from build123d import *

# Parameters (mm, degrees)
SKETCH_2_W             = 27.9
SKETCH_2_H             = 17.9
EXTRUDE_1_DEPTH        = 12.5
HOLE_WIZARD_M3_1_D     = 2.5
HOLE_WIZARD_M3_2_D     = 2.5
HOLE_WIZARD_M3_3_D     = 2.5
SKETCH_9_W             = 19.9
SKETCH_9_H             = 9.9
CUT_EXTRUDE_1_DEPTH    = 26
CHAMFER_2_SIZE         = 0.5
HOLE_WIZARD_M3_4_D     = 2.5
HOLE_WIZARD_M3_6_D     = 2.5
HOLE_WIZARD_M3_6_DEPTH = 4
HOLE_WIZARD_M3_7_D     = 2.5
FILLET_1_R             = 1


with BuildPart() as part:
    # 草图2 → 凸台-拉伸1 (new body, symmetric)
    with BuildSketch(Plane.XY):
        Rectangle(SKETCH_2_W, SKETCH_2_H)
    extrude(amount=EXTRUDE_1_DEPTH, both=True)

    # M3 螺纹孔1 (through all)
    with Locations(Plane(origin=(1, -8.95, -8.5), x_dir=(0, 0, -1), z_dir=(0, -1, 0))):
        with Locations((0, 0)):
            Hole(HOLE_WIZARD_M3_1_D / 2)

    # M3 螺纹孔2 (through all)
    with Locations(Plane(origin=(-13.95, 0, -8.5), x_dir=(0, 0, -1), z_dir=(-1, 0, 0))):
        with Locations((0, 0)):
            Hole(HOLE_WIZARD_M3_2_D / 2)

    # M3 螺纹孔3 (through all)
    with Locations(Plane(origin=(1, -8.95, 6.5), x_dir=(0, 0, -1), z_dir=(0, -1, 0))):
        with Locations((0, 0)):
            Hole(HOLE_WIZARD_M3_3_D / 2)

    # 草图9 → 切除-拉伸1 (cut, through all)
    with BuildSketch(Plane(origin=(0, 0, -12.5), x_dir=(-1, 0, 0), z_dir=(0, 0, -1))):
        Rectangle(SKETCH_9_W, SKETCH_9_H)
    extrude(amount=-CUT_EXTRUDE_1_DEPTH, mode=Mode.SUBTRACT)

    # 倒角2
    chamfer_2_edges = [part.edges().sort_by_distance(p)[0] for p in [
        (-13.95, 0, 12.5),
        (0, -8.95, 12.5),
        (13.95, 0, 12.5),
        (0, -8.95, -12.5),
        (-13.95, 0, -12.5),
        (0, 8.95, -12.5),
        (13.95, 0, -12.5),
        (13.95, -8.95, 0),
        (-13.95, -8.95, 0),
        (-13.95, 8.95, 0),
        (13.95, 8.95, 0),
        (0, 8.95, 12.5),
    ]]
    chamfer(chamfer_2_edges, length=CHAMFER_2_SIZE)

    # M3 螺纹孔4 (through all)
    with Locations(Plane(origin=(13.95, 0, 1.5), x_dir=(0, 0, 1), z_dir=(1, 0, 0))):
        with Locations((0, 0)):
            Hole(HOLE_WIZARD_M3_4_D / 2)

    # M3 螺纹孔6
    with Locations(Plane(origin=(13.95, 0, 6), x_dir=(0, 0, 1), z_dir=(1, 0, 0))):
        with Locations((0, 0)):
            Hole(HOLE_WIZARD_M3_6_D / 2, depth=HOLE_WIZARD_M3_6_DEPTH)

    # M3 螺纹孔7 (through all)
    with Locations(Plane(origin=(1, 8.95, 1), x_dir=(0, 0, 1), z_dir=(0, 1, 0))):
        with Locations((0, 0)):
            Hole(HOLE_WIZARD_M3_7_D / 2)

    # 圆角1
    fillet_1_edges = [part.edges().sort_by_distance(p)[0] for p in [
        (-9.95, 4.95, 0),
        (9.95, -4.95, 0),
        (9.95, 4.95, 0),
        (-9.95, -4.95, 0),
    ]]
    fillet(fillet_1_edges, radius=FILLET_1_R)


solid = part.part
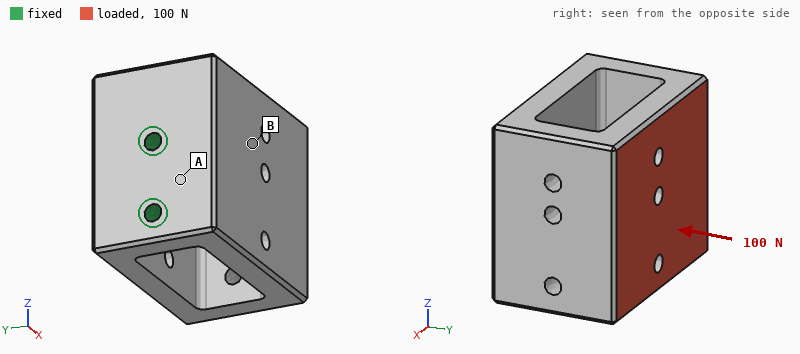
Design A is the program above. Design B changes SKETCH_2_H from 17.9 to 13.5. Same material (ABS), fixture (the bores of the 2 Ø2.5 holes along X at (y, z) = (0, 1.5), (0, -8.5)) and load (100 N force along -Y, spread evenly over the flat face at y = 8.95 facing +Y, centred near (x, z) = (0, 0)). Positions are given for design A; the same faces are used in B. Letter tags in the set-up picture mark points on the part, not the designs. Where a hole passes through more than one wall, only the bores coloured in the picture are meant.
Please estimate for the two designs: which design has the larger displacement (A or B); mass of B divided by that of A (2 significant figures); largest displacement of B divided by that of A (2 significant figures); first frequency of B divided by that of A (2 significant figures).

B
0.59
2.4
0.81
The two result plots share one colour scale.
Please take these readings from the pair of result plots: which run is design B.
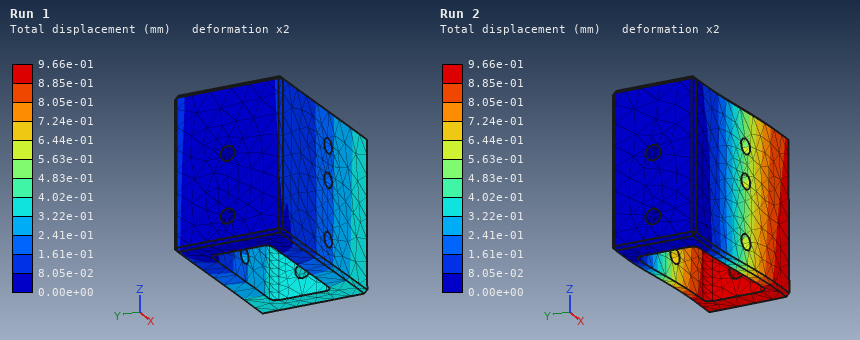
Run 2
